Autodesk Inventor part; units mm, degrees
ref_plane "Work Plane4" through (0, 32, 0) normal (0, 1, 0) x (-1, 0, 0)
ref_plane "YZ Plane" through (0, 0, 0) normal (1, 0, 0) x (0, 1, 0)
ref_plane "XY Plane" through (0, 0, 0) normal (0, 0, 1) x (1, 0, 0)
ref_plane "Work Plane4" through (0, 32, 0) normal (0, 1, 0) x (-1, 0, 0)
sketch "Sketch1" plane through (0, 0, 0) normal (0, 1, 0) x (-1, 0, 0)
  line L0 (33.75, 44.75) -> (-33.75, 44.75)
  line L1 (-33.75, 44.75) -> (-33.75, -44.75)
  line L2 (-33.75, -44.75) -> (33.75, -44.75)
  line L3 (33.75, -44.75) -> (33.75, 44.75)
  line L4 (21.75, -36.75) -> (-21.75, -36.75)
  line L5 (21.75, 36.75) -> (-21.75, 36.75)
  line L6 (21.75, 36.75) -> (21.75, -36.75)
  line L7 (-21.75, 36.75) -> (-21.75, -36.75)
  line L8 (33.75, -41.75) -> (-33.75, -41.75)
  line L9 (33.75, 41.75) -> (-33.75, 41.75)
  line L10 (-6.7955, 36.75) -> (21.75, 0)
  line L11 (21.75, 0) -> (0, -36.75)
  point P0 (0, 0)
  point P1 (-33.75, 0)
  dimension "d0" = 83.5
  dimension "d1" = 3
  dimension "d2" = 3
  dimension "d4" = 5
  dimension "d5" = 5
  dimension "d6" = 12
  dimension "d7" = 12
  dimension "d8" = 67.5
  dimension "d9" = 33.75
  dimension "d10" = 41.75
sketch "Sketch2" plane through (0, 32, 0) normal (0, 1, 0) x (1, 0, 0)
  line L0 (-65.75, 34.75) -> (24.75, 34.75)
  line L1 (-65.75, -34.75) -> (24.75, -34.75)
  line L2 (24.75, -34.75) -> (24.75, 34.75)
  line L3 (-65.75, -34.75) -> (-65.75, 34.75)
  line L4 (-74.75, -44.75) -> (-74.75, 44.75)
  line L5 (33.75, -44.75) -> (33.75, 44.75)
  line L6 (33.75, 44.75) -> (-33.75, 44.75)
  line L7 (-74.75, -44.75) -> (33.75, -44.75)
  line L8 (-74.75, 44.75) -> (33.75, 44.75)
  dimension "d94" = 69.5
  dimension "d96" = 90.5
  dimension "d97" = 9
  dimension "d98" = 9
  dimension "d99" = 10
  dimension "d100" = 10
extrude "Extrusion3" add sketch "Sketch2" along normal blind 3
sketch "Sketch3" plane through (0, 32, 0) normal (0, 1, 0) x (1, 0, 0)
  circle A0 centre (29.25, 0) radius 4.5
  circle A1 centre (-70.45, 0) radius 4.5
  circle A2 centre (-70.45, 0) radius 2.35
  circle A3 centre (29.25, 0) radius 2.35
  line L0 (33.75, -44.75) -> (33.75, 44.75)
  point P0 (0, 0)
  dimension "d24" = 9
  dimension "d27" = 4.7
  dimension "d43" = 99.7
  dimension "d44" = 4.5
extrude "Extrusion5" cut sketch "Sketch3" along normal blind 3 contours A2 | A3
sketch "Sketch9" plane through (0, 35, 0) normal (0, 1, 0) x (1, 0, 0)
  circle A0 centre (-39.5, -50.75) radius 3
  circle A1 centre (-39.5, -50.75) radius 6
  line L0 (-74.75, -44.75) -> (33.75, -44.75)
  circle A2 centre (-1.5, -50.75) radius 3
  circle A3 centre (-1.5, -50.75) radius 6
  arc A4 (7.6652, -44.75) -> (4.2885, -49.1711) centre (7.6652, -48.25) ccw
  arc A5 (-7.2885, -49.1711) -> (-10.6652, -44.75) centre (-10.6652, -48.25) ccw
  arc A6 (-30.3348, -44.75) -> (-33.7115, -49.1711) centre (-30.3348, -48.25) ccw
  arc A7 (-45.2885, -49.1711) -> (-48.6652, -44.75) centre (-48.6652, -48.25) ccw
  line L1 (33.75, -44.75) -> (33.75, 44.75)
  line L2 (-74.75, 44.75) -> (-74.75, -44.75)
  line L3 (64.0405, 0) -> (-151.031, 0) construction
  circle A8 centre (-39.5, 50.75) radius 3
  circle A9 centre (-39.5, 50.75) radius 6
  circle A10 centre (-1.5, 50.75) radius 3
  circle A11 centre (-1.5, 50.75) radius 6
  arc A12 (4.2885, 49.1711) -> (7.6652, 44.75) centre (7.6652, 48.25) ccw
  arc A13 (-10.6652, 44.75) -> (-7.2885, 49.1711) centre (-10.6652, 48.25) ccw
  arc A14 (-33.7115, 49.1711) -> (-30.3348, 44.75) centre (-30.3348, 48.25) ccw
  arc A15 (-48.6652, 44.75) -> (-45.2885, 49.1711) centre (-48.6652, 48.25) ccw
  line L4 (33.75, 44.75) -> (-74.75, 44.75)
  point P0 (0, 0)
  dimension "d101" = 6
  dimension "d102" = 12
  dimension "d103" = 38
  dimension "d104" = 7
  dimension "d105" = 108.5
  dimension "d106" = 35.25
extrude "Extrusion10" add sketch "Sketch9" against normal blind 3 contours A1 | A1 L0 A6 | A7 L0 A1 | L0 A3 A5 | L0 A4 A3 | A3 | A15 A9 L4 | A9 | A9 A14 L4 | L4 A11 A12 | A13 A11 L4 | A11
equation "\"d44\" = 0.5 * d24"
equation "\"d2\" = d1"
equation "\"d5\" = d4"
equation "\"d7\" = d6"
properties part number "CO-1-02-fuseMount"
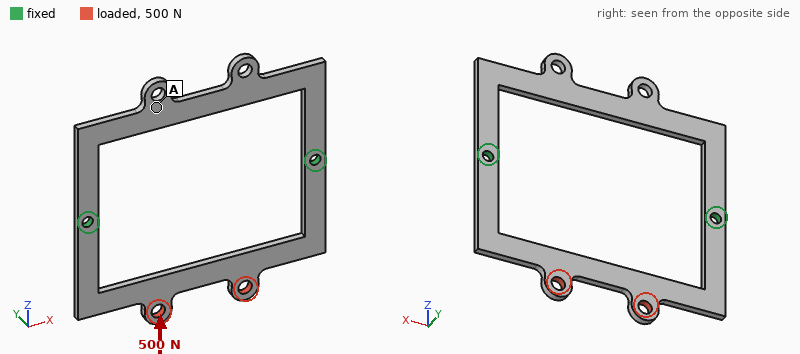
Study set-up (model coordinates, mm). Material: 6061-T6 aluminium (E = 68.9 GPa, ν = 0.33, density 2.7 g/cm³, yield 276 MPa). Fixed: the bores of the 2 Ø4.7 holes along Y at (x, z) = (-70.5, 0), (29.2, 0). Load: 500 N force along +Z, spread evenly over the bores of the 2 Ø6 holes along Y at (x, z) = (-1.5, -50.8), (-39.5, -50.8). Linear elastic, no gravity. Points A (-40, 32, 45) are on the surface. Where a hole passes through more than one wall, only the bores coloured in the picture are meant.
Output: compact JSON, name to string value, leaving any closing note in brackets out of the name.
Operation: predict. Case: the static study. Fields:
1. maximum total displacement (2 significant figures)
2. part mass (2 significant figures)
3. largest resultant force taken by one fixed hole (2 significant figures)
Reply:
{"maximum total displacement": "0.17 mm", "part mass": "31 g", "largest resultant force taken by one fixed hole": "290 N"}
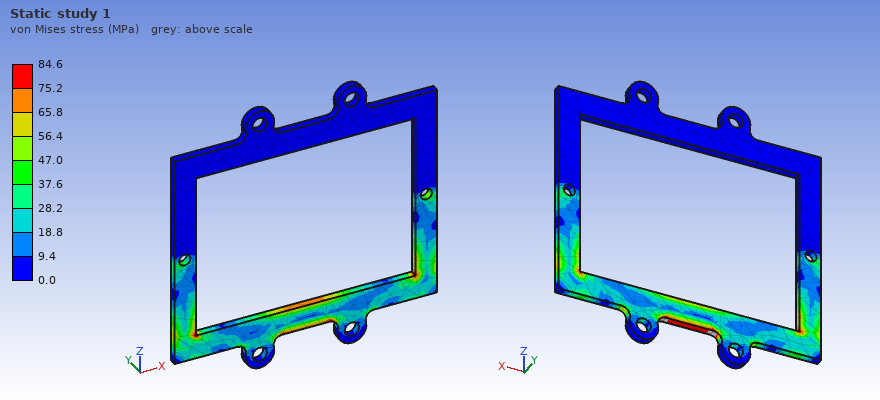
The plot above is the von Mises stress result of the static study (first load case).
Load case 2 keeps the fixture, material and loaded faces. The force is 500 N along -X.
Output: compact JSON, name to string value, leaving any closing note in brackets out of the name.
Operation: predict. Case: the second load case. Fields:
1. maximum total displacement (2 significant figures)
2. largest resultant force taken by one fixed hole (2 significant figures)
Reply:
{"maximum total displacement": "0.18 mm", "largest resultant force taken by one fixed hole": "290 N"}
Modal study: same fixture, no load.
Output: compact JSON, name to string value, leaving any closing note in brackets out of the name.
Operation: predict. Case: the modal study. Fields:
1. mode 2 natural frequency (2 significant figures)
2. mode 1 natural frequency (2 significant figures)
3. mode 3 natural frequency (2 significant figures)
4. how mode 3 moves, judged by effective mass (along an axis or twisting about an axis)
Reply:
{"mode 2 natural frequency": "480 Hz", "mode 1 natural frequency": "480 Hz", "mode 3 natural frequency": "1100 Hz", "how mode 3 moves, judged by effective mass": "twisting about Z"}
